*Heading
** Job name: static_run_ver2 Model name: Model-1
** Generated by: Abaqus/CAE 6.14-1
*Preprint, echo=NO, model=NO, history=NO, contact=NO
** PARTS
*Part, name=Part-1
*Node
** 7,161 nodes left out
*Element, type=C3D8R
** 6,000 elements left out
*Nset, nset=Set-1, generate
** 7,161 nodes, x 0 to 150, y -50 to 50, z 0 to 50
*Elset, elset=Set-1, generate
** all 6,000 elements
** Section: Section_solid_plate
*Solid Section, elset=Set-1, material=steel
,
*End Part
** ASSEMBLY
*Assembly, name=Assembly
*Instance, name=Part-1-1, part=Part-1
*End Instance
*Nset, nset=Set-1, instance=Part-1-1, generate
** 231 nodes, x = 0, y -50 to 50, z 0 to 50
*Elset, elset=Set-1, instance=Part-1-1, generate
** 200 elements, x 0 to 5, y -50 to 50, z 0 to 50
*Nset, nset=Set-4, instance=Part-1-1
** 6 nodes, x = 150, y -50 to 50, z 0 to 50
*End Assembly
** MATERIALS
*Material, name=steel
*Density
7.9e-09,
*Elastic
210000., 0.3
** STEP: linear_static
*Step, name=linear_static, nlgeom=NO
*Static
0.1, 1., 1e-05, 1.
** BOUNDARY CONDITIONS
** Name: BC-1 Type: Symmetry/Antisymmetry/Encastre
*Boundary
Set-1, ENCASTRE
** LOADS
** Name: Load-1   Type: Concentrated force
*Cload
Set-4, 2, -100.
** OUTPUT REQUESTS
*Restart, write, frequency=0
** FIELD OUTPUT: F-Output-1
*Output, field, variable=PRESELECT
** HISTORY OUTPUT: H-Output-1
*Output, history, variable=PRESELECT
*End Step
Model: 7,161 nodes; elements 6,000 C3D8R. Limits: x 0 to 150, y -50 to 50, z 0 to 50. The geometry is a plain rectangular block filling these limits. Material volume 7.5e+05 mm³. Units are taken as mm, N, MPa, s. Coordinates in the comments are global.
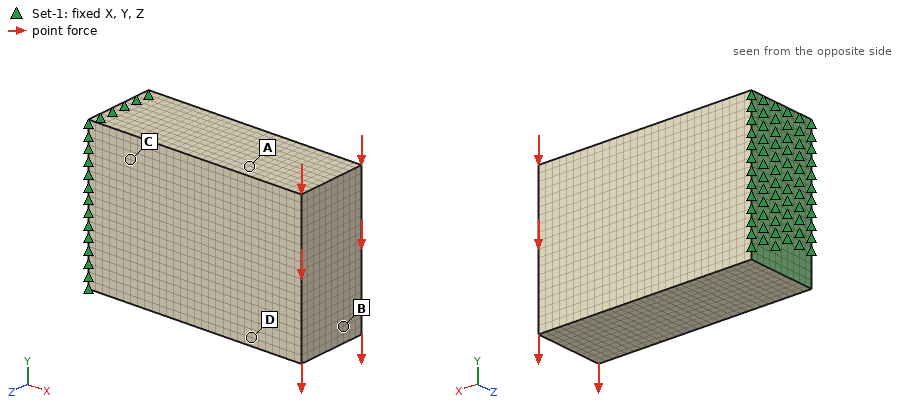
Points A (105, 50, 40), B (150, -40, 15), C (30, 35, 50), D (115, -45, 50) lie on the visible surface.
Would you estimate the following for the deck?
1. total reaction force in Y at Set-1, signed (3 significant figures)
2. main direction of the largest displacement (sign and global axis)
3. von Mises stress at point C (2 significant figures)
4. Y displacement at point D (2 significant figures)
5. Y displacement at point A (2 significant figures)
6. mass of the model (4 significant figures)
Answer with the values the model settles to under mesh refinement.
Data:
600 N
-Y
0.61 MPa
-6.9e-04 mm
-6.1e-04 mm
5.925 kg
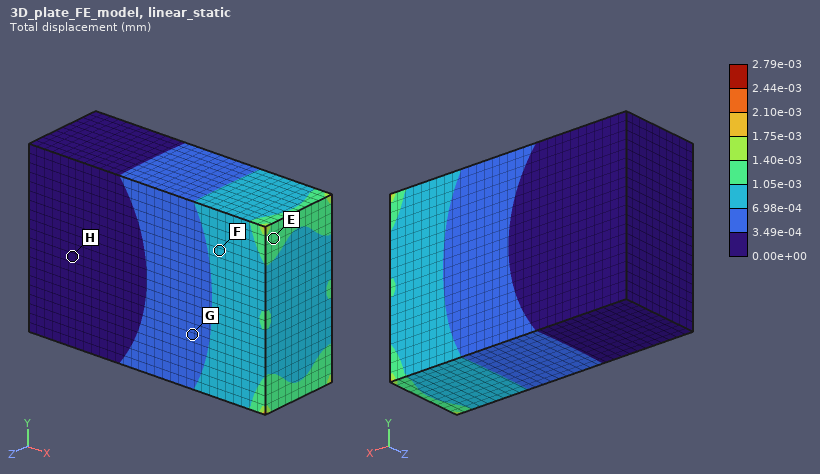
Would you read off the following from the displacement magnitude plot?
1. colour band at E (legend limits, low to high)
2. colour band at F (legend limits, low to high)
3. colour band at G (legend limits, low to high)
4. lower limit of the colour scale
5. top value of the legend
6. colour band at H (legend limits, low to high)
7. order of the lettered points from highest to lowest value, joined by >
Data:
1.05e-03 to 1.40e-03 mm
6.98e-04 to 1.05e-03 mm
3.49e-04 to 6.98e-04 mm
0.00e+00 mm
2.79e-03 mm
0.00e+00 to 3.49e-04 mm
E > F > G > H
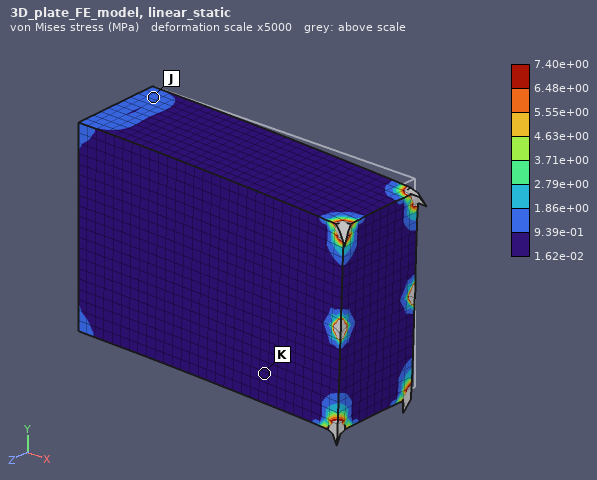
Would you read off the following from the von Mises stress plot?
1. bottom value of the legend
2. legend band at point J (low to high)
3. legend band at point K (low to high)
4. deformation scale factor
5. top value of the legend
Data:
1.62e-02 MPa
9.39e-01 to 1.86e+00 MPa
1.62e-02 to 9.39e-01 MPa
5000
7.40e+00 MPa
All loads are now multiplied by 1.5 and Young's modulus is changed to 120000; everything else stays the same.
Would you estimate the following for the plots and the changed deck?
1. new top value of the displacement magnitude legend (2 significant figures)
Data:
0.0073 mm
